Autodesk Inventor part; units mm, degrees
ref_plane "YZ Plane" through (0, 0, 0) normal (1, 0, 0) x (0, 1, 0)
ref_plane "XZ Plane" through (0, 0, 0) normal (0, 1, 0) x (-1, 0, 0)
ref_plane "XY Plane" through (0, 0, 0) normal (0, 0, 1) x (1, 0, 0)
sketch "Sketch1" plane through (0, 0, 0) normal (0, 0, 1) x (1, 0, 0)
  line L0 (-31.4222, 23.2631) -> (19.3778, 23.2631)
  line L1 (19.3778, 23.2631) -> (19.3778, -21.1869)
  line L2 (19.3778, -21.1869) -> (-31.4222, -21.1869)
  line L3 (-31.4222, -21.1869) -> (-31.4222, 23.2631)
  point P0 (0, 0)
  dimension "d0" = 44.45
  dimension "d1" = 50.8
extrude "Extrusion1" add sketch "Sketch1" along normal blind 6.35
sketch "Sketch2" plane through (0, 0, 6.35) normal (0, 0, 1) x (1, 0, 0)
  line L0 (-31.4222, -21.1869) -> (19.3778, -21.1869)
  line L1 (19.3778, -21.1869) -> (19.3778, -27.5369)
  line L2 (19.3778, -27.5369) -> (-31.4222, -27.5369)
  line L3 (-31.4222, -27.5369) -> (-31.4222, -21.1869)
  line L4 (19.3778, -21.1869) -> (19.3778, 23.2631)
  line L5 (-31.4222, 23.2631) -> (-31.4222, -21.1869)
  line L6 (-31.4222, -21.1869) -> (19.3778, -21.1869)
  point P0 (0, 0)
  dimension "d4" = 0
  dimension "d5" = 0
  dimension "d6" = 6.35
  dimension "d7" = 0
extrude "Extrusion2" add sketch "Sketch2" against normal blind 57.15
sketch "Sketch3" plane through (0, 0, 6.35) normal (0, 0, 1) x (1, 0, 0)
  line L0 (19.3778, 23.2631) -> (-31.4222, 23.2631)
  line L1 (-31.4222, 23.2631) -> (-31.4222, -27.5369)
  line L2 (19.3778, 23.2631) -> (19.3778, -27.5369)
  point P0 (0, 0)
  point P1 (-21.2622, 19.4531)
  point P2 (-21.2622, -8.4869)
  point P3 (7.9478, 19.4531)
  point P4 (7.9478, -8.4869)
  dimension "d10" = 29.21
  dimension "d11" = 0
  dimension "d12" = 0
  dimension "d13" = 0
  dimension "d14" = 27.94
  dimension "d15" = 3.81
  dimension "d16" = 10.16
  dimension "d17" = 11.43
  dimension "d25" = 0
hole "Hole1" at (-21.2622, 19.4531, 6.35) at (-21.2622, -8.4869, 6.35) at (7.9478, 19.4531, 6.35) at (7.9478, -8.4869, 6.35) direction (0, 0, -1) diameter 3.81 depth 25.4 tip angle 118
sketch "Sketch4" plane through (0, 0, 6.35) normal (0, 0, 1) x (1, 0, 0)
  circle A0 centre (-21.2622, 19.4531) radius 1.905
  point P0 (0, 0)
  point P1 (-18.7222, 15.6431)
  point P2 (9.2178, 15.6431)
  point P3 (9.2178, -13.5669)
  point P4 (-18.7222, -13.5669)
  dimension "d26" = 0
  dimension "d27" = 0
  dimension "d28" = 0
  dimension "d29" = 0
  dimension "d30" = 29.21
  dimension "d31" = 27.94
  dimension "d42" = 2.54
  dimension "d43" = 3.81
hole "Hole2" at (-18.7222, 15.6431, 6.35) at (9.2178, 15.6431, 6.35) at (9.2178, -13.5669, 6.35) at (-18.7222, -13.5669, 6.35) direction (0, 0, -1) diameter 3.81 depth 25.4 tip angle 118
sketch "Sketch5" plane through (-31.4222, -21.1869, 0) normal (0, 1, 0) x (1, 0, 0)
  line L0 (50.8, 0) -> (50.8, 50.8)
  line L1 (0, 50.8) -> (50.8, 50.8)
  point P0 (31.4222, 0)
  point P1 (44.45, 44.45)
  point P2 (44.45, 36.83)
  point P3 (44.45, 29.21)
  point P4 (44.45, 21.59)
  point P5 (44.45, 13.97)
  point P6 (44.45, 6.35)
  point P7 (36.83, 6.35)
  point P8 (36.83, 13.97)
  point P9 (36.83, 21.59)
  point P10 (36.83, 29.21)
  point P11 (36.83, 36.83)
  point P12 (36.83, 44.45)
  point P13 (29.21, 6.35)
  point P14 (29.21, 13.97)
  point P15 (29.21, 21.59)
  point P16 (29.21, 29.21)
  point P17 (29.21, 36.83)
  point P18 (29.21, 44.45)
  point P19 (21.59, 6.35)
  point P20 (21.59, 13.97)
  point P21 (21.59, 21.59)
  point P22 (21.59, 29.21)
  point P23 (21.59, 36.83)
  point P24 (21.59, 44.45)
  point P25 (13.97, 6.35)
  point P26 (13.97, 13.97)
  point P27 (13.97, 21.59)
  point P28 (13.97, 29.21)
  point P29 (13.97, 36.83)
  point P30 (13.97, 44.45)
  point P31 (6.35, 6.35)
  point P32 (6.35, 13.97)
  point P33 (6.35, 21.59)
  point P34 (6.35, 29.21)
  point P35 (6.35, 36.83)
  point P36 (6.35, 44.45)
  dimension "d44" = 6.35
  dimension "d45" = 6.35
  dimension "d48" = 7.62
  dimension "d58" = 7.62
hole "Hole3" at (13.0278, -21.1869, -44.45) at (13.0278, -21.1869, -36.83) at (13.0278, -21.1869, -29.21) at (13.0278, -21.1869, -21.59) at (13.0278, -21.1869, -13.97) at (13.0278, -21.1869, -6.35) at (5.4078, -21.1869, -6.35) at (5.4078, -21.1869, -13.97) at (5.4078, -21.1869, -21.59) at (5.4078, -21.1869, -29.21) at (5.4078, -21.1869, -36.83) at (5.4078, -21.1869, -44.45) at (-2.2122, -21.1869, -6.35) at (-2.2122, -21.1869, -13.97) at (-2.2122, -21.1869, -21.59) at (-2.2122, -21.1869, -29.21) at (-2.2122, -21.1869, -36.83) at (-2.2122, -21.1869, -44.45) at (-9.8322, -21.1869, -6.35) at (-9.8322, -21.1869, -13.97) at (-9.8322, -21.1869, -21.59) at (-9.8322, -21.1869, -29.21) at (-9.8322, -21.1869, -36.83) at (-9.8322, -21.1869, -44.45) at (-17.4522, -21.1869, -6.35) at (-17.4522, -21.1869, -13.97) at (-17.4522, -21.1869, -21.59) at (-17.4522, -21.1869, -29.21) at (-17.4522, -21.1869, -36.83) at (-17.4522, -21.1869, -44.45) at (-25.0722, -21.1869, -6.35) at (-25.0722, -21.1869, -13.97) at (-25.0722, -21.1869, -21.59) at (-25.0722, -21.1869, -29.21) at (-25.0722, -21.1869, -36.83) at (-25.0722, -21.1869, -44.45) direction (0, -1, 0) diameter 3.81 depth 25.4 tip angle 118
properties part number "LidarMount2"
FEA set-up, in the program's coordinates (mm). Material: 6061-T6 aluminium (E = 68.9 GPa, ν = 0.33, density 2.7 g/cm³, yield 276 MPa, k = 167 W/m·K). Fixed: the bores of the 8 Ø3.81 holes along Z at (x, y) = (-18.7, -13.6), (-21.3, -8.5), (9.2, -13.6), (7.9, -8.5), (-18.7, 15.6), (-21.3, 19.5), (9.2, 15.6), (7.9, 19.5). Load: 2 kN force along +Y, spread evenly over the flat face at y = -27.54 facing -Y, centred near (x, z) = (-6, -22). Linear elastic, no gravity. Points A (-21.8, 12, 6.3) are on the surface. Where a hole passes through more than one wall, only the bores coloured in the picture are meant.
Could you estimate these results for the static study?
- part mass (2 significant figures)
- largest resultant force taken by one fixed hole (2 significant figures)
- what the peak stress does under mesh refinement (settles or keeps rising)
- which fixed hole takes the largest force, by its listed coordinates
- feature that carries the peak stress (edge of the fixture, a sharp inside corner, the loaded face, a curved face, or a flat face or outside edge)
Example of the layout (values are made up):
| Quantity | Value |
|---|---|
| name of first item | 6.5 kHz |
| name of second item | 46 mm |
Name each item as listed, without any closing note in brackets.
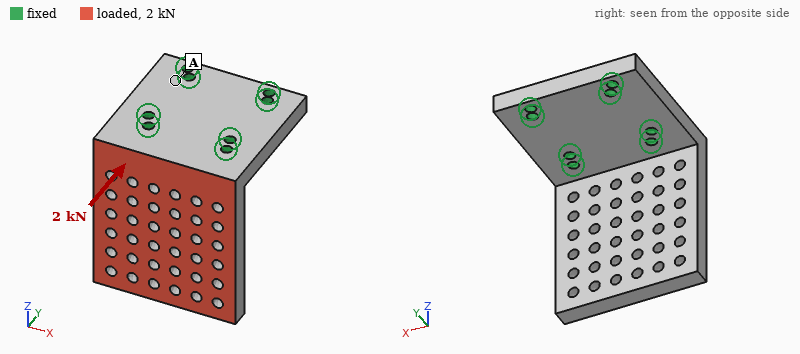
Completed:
| Quantity | Value |
|---|---|
| part mass | 80 g |
| largest resultant force taken by one fixed hole | 1.4 kN |
| what the peak stress does under mesh refinement | keeps rising |
| which fixed hole takes the largest force, by its listed coordinates | (-18.7, -13.6) |
| feature that carries the peak stress | edge of the fixture |
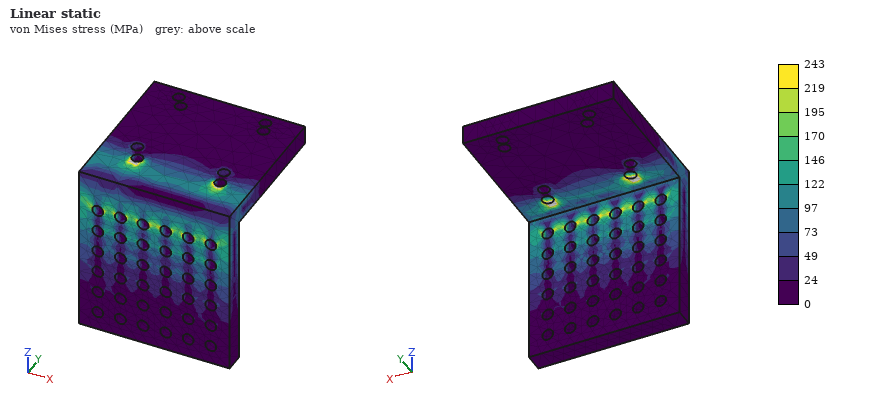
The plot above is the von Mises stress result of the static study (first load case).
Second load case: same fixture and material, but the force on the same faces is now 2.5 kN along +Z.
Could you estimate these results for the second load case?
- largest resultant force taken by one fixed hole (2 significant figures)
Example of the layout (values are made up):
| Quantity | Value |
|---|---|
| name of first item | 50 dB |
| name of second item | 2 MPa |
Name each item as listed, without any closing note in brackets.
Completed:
| Quantity | Value |
|---|---|
| largest resultant force taken by one fixed hole | 1.8 kN |
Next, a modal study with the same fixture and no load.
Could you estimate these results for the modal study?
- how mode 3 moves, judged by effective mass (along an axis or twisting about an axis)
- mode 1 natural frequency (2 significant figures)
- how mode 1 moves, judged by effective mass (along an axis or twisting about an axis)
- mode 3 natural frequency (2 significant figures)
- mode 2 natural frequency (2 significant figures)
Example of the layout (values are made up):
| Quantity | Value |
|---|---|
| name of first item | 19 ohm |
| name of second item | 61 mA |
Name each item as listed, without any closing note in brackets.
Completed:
| Quantity | Value |
|---|---|
| how mode 3 moves, judged by effective mass | along X |
| mode 1 natural frequency | 1400 Hz |
| how mode 1 moves, judged by effective mass | along Y |
| mode 3 natural frequency | 4500 Hz |
| mode 2 natural frequency | 3300 Hz |
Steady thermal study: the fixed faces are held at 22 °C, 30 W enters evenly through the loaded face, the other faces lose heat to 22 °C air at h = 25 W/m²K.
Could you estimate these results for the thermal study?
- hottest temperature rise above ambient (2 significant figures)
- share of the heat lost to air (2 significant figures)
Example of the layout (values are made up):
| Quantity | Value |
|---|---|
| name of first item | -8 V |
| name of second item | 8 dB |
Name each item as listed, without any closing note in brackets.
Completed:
| Quantity | Value |
|---|---|
| hottest temperature rise above ambient | 22 K |
| share of the heat lost to air | 8.8 % |
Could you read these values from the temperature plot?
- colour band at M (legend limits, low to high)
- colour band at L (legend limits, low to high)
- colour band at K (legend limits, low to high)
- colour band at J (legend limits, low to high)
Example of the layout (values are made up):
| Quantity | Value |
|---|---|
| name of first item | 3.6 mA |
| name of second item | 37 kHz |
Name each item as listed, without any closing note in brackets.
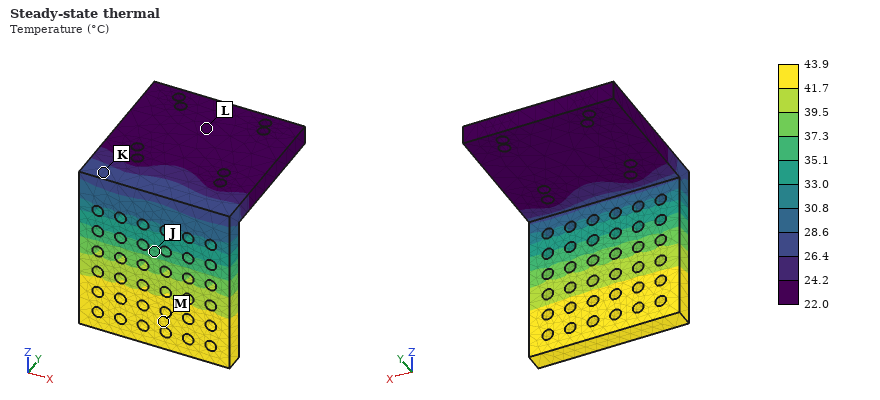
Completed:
| Quantity | Value |
|---|---|
| colour band at M | 41.7 to 43.9 °C |
| colour band at L | 22.0 to 24.2 °C |
| colour band at K | 26.4 to 28.6 °C |
| colour band at J | 35.1 to 37.3 °C |
